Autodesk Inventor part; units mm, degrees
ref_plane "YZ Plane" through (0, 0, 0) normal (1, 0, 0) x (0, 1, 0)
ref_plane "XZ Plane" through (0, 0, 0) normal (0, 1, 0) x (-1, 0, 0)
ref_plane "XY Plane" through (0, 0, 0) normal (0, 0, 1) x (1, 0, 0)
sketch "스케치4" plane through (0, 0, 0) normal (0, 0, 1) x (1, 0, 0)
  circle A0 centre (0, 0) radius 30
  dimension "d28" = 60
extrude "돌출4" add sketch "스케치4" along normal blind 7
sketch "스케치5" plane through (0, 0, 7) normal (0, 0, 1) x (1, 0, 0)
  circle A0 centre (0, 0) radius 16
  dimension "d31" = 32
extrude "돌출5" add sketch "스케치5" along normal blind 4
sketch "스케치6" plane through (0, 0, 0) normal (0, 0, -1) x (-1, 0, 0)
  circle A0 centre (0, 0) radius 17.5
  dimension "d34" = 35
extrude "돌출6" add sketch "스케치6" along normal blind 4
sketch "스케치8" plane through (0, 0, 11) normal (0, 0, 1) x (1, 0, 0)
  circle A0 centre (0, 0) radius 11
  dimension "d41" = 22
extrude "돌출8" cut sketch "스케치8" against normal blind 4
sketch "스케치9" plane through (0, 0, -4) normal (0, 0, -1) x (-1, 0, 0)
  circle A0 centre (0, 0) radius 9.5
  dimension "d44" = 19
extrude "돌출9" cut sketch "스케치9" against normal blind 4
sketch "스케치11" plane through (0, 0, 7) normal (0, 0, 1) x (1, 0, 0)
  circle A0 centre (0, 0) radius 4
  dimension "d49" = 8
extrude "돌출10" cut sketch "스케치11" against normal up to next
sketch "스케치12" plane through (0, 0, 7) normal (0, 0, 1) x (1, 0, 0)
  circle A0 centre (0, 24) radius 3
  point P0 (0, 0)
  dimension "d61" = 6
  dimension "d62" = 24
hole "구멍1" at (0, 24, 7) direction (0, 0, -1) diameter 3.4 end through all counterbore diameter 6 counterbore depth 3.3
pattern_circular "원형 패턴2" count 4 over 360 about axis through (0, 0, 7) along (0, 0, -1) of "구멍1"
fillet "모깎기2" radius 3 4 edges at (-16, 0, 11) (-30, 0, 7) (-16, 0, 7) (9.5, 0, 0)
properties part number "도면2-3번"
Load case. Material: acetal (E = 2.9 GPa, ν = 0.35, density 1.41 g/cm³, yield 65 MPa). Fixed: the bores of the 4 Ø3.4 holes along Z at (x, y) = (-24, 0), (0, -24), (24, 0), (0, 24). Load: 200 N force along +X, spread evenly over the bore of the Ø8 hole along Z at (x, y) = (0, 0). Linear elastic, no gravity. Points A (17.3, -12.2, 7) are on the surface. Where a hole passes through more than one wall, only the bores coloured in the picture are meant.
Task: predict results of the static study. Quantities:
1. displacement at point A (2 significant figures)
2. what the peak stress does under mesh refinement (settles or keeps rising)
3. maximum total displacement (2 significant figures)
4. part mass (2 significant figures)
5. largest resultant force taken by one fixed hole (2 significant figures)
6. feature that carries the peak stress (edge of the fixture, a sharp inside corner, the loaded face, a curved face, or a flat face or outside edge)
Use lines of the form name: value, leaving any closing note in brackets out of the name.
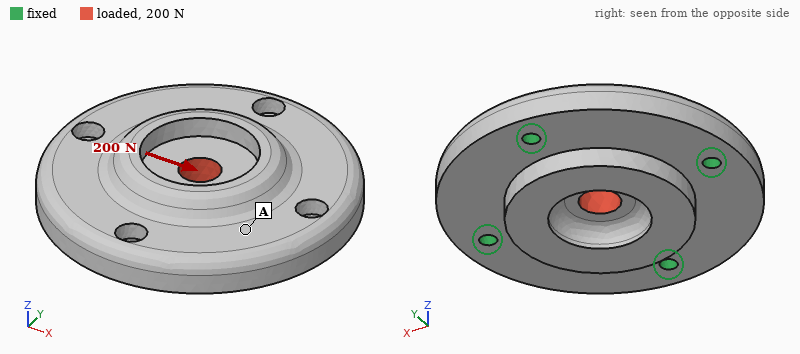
displacement at point A: 3.4 µm
what the peak stress does under mesh refinement: keeps rising
maximum total displacement: 6.9 µm
part mass: 32 g
largest resultant force taken by one fixed hole: 62 N
feature that carries the peak stress: edge of the fixture
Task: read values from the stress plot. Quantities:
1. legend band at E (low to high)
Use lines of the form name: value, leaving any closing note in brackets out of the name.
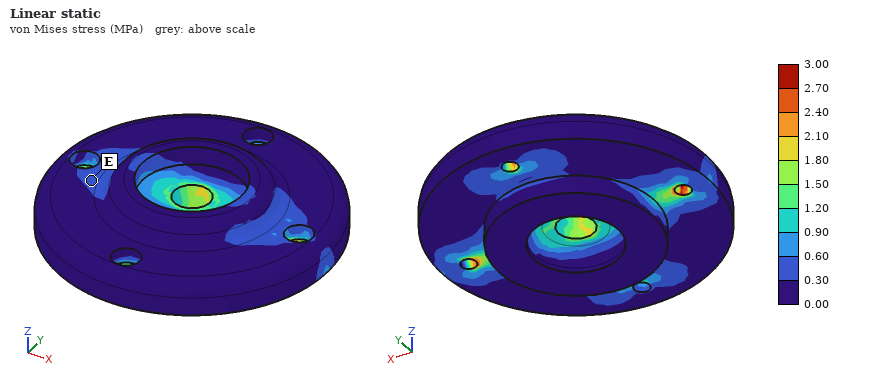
legend band at E: 0.30 to 0.60 MPa
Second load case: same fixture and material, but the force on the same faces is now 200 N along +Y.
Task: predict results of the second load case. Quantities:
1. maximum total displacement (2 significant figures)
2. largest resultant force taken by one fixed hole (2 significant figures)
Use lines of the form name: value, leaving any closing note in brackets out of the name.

maximum total displacement: 6.9 µm
largest resultant force taken by one fixed hole: 62 N
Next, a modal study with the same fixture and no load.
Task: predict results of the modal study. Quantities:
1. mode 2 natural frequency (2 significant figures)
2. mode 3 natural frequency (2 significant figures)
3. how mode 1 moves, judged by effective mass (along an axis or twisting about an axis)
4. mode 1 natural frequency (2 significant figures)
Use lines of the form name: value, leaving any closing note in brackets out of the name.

mode 2 natural frequency: 4700 Hz
mode 3 natural frequency: 5000 Hz
how mode 1 moves, judged by effective mass: along Z
mode 1 natural frequency: 4500 Hz
